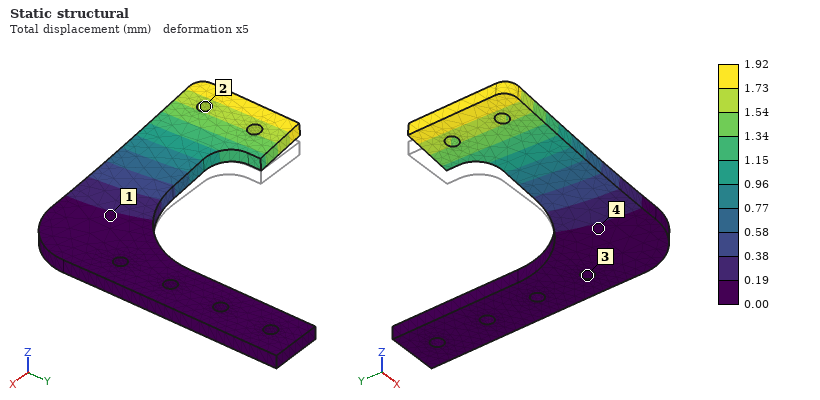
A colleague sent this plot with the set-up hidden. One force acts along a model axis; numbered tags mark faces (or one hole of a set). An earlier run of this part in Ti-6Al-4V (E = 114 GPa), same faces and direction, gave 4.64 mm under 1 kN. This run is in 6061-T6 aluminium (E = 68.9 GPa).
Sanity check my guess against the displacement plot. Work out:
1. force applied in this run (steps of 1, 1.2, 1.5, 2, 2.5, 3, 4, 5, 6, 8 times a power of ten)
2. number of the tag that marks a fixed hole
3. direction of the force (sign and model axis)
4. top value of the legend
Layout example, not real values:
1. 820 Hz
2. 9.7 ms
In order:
1. 250 N
2. 3
3. +Z
4. 1.92 mm
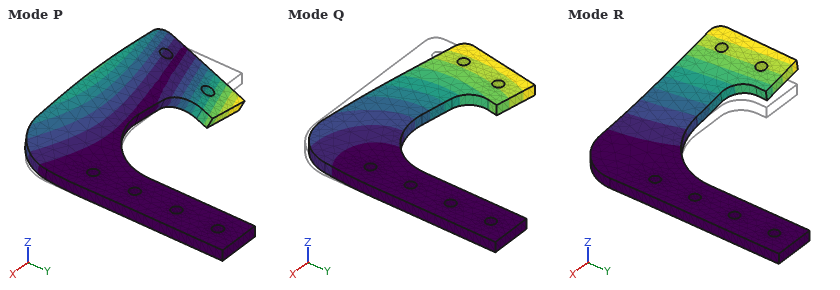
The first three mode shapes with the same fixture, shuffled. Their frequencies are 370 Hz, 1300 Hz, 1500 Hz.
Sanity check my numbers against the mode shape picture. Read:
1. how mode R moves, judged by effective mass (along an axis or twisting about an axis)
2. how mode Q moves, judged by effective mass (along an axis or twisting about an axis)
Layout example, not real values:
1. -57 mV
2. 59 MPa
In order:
1. along Z
2. along Y
